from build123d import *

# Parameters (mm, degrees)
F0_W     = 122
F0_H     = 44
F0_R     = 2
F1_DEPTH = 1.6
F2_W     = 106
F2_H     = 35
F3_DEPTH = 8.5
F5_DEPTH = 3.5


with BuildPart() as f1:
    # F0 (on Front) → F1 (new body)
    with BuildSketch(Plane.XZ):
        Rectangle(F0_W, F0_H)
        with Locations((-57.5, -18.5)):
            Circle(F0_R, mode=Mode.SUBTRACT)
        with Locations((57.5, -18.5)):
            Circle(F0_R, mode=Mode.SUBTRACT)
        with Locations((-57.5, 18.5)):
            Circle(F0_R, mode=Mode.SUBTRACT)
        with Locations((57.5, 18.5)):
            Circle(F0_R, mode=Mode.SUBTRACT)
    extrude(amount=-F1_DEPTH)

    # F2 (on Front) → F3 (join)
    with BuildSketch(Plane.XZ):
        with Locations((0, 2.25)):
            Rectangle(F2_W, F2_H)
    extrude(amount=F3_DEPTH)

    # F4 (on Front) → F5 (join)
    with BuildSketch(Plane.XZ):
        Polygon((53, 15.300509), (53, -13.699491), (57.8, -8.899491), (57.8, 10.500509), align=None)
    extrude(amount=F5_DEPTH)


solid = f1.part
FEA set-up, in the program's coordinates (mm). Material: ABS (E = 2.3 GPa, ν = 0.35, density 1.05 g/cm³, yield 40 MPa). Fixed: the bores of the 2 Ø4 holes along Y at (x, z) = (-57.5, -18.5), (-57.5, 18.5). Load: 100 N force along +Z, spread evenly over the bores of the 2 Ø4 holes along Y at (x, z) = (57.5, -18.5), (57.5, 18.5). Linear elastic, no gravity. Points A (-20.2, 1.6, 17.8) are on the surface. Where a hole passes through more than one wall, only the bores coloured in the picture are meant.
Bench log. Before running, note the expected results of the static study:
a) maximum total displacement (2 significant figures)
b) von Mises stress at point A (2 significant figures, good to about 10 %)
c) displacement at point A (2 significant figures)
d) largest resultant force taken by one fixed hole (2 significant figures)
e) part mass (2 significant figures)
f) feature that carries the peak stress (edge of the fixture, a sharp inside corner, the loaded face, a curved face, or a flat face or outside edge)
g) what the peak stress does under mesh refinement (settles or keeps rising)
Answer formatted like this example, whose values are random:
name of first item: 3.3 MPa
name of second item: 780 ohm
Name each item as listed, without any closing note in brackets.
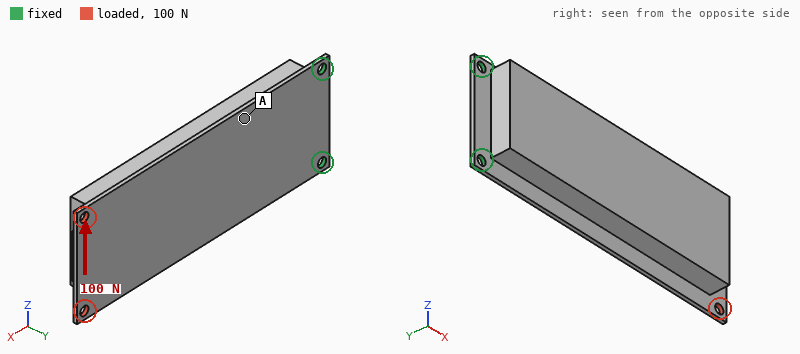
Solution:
maximum total displacement: 1.3 mm
von Mises stress at point A: 3.5 MPa
displacement at point A: 0.30 mm
largest resultant force taken by one fixed hole: 320 N
part mass: 42 g
feature that carries the peak stress: edge of the fixture
what the peak stress does under mesh refinement: keeps rising
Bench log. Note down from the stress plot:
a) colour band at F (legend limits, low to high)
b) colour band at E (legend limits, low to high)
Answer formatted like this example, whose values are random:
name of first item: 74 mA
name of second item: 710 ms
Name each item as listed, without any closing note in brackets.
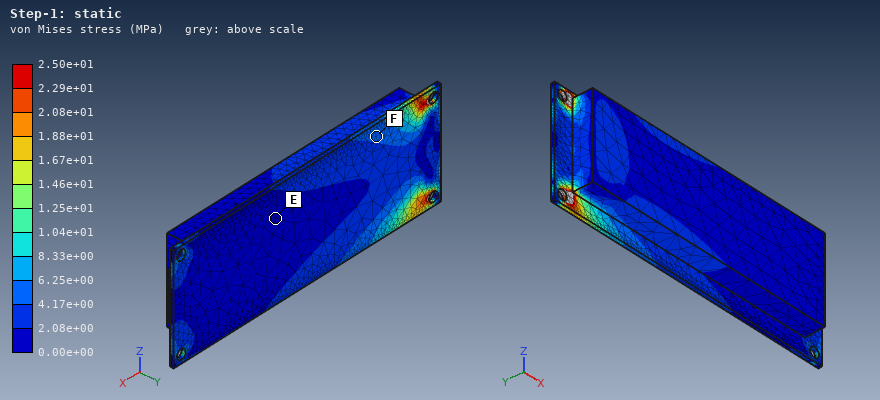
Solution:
colour band at F: 4.17e+00 to 6.25e+00 MPa
colour band at E: 0.00e+00 to 2.08e+00 MPa
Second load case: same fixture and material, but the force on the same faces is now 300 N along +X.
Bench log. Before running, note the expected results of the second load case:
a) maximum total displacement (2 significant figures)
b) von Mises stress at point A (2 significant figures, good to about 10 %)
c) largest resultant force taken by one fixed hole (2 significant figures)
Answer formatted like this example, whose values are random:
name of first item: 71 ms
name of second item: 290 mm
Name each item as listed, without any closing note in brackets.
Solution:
maximum total displacement: 1.3 mm
von Mises stress at point A: 2.5 MPa
largest resultant force taken by one fixed hole: 160 N
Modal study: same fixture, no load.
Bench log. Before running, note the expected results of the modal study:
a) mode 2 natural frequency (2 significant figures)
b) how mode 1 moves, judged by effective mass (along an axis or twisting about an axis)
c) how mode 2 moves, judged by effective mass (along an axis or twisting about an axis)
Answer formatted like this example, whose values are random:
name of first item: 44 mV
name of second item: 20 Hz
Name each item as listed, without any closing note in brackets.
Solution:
mode 2 natural frequency: 440 Hz
how mode 1 moves, judged by effective mass: along Y
how mode 2 moves, judged by effective mass: along Z
